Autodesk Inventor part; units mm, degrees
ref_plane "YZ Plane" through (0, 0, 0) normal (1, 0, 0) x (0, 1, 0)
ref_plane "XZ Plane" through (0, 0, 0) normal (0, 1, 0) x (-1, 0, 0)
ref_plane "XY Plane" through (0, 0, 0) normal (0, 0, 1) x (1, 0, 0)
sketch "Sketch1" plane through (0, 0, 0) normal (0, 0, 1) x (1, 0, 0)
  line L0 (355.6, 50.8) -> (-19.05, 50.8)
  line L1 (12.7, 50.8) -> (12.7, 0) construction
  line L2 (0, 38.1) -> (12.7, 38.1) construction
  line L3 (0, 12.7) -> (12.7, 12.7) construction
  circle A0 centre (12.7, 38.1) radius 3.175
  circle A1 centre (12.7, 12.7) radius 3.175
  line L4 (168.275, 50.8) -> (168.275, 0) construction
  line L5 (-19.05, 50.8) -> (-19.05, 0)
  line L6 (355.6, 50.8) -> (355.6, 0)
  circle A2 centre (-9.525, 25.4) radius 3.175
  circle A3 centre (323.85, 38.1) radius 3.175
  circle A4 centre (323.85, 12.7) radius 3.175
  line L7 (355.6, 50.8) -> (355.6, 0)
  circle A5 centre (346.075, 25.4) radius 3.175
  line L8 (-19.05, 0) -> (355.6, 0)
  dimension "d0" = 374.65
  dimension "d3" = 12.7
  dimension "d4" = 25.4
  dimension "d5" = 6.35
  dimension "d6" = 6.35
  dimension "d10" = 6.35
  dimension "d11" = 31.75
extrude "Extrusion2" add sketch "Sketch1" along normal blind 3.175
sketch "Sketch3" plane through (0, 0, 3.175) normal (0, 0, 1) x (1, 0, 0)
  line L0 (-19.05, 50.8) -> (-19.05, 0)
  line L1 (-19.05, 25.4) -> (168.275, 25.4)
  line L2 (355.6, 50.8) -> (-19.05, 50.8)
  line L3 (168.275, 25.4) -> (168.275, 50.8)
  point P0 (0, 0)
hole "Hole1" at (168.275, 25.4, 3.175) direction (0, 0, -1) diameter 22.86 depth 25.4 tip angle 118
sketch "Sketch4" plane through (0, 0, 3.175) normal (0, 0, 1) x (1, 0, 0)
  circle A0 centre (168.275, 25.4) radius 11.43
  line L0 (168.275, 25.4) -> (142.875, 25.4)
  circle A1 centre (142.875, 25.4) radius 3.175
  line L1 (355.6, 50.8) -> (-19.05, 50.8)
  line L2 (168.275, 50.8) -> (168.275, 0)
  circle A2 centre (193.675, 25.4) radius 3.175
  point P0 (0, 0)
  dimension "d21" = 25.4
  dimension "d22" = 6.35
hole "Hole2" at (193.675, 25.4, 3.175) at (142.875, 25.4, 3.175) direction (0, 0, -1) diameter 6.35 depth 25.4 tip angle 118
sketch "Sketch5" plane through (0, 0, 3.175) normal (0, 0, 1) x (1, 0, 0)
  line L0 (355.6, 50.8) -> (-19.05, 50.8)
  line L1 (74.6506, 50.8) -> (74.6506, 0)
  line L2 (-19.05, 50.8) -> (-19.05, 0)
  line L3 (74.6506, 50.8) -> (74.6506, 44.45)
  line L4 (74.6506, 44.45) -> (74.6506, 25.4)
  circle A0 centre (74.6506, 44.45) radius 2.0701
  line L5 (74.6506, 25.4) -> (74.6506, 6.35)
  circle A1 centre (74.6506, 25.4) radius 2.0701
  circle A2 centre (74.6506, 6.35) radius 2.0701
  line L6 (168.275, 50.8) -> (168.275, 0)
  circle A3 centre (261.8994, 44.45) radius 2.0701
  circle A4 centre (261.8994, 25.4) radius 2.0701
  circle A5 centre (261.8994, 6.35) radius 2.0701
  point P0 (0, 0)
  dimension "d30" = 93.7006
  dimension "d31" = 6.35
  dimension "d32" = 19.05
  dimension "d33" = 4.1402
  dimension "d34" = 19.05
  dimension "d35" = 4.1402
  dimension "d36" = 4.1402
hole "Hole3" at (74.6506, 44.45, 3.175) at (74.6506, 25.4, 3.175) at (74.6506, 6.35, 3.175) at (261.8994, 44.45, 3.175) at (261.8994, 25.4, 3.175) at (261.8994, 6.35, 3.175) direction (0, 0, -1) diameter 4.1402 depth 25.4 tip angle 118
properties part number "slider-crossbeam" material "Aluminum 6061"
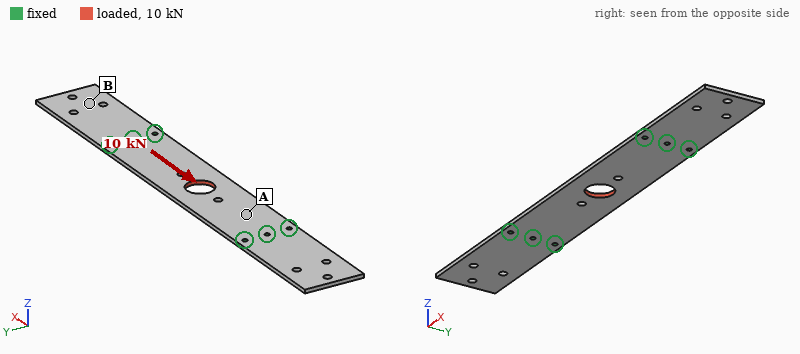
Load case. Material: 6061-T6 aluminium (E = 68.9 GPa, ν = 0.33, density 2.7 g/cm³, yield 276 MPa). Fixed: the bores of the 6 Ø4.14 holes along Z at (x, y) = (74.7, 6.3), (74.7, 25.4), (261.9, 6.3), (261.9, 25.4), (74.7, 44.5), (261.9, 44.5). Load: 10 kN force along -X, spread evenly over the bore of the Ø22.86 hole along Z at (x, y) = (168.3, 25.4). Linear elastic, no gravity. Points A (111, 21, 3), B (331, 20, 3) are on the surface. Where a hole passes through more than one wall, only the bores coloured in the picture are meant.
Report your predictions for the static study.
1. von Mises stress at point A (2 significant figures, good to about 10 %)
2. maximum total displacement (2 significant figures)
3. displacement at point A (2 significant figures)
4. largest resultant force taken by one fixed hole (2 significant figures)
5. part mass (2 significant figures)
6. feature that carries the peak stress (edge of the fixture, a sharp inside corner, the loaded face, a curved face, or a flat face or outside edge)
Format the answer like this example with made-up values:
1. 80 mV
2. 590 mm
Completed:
1. 31 MPa
2. 46 µm
3. 17 µm
4. 1.7 kN
5. 160 g
6. a curved face
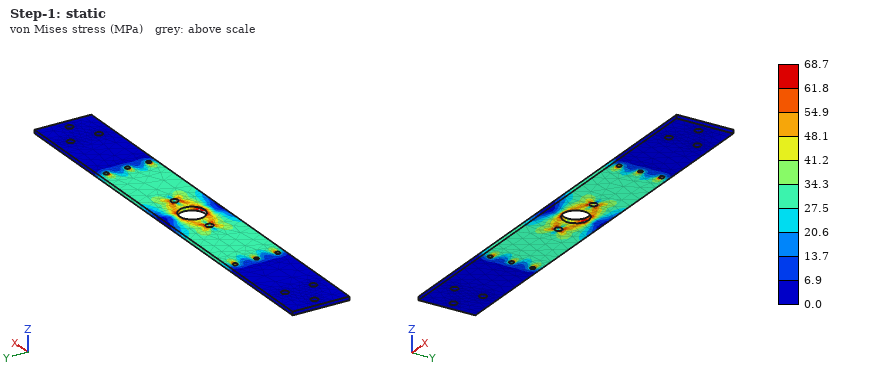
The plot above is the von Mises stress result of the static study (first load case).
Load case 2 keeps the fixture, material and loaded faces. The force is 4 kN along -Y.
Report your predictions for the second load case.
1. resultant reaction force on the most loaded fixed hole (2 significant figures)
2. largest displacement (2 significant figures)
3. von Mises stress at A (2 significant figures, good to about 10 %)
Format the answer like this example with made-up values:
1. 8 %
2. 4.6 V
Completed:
1. 2.4 kN
2. 0.11 mm
3. 32 MPa
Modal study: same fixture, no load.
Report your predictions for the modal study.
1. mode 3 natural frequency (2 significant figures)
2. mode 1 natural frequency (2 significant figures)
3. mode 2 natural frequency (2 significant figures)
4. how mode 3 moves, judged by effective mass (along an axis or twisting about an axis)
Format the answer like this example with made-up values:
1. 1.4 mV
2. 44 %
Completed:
1. 490 Hz
2. 310 Hz
3. 310 Hz
4. along Z
